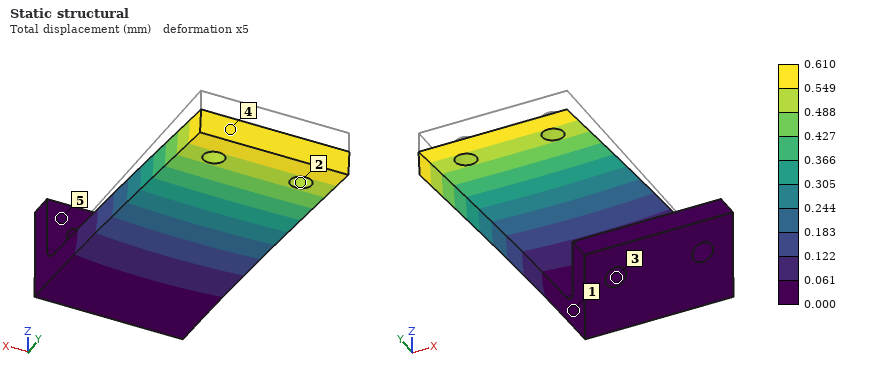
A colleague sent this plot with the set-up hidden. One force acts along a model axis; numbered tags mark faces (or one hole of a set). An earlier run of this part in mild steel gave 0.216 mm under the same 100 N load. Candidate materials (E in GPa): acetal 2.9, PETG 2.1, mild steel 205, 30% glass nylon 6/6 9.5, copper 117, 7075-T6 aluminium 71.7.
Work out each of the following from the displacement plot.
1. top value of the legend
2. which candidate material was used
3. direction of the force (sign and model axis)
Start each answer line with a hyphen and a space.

- 0.610 mm
- 7075-T6 aluminium
- -Z
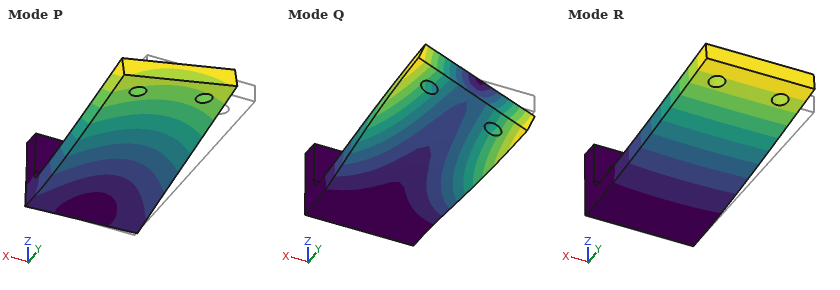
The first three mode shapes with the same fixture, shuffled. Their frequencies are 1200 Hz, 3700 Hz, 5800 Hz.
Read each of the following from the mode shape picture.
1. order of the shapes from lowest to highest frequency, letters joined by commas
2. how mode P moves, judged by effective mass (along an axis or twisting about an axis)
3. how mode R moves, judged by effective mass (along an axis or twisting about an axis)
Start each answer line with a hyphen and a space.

- R, P, Q
- along X
- along Z
